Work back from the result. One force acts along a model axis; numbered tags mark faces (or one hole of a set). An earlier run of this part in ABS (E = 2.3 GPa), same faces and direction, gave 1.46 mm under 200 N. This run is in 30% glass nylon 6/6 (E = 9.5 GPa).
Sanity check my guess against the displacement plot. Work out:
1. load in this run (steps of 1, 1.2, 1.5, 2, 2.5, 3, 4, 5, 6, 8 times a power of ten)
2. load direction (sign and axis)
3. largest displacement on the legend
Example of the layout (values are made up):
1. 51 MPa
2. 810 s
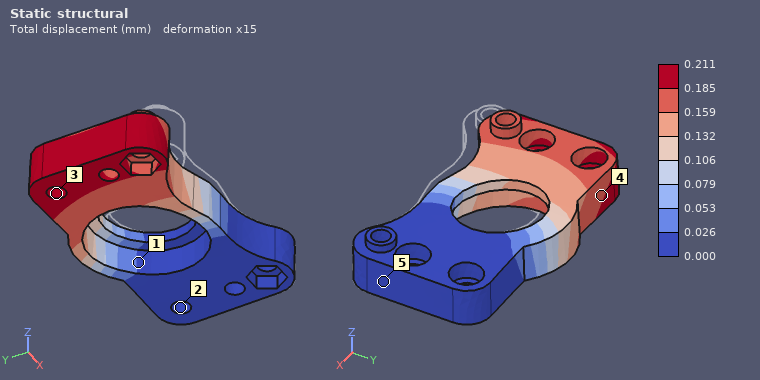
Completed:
1. 120 N
2. +Y
3. 0.211 mm
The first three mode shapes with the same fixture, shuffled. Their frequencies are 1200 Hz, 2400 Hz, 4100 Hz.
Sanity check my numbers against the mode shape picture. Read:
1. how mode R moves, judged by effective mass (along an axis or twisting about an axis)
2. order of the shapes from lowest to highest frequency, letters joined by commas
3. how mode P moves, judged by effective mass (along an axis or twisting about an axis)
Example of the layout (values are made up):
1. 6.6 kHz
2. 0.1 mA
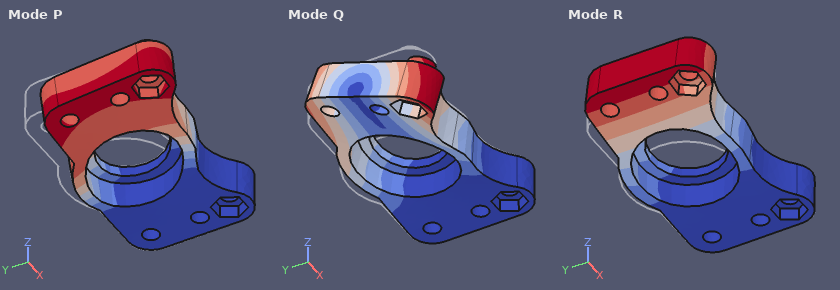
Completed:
1. along Z
2. R, P, Q
3. along Y
